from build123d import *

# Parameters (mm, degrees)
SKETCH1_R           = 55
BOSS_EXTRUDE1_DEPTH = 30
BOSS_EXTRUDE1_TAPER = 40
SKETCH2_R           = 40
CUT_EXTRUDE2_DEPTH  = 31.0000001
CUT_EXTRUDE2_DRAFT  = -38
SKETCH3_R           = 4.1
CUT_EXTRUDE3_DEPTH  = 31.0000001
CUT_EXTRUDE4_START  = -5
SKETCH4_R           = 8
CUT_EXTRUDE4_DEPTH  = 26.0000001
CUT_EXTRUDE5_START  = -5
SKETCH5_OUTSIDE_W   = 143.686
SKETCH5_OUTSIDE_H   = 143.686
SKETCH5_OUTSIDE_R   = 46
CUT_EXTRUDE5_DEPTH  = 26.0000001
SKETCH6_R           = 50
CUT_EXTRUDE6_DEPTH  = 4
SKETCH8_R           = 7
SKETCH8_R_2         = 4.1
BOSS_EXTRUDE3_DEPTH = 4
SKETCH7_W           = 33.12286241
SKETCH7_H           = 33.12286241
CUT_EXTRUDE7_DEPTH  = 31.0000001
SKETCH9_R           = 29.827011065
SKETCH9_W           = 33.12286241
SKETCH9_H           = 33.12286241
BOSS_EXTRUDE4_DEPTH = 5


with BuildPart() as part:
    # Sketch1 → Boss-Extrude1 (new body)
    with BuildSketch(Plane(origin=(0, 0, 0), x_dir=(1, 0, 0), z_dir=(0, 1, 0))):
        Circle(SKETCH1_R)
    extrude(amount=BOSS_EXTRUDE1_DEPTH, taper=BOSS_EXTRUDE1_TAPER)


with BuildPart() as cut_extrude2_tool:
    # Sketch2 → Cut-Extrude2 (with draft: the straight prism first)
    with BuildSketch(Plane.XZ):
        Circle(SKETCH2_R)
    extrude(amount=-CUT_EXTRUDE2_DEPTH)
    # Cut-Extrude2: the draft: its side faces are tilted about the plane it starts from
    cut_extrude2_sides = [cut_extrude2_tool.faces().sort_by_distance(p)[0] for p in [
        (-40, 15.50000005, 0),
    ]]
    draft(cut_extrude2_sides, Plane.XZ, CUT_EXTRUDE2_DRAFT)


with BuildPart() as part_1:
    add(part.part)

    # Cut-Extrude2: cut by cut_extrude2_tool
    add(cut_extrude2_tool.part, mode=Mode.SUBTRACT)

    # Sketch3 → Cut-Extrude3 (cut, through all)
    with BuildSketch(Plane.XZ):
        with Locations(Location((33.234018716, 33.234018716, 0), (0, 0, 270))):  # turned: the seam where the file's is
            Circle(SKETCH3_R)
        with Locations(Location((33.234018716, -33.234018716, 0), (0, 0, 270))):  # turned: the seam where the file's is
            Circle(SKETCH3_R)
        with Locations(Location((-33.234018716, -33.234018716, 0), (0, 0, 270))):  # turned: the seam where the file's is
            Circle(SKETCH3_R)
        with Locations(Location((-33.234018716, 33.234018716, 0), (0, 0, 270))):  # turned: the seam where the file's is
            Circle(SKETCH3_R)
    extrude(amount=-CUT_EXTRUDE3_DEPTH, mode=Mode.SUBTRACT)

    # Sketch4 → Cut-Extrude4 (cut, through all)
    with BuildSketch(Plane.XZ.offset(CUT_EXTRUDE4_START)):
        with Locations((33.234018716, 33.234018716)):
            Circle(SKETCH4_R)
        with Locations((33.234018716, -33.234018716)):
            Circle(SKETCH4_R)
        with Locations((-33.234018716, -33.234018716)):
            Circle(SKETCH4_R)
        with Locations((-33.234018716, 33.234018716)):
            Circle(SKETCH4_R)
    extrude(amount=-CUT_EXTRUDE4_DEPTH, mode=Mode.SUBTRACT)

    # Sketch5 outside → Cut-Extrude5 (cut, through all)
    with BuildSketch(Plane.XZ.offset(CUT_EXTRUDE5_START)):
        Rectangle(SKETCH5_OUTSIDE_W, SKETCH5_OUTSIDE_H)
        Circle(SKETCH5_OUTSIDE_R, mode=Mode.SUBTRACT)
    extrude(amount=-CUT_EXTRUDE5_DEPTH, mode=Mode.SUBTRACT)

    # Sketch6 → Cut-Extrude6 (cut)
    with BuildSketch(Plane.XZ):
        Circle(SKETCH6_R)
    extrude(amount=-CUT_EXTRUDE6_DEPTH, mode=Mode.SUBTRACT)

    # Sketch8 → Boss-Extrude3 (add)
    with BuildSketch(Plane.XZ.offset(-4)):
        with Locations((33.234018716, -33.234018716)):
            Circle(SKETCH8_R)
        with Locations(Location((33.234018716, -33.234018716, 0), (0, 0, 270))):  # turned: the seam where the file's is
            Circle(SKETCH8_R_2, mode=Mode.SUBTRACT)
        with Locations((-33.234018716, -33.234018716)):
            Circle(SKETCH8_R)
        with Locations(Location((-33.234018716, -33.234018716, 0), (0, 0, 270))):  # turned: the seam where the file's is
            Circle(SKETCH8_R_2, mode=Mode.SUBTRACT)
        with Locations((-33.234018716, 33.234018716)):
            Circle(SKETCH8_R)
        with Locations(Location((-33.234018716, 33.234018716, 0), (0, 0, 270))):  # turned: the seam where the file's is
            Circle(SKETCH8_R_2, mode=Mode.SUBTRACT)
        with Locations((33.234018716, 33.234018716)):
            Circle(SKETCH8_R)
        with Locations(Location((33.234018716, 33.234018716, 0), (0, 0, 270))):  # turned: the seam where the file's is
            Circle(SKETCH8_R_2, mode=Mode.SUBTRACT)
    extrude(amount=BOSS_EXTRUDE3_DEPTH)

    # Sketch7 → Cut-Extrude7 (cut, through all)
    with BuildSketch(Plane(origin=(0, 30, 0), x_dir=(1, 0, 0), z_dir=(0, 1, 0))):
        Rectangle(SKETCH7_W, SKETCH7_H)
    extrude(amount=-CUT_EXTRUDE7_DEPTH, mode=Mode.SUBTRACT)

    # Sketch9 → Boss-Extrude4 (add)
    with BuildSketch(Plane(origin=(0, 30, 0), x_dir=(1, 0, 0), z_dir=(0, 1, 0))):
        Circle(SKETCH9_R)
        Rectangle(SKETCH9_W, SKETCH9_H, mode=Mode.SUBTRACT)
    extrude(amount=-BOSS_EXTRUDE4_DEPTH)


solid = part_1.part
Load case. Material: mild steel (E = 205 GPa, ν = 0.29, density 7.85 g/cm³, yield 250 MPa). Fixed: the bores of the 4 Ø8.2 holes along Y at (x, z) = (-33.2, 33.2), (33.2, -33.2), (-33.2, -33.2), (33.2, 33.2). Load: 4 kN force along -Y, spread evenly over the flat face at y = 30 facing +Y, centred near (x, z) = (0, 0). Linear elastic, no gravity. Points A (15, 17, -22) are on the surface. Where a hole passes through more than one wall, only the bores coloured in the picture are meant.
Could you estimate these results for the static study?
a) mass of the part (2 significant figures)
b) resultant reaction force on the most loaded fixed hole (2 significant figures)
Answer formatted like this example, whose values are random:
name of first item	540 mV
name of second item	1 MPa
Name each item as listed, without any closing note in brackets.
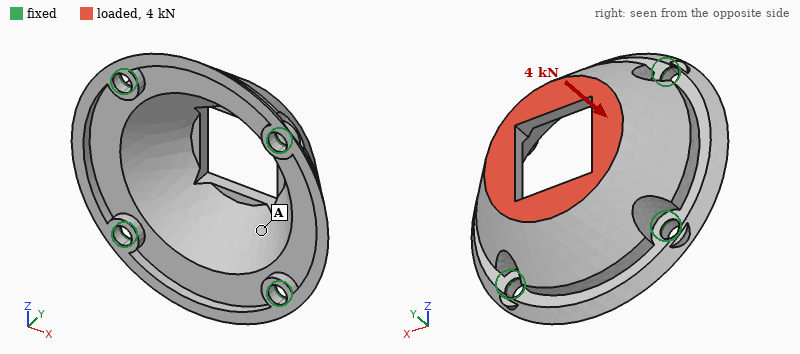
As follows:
mass of the part	590 g
resultant reaction force on the most loaded fixed hole	1.3 kN
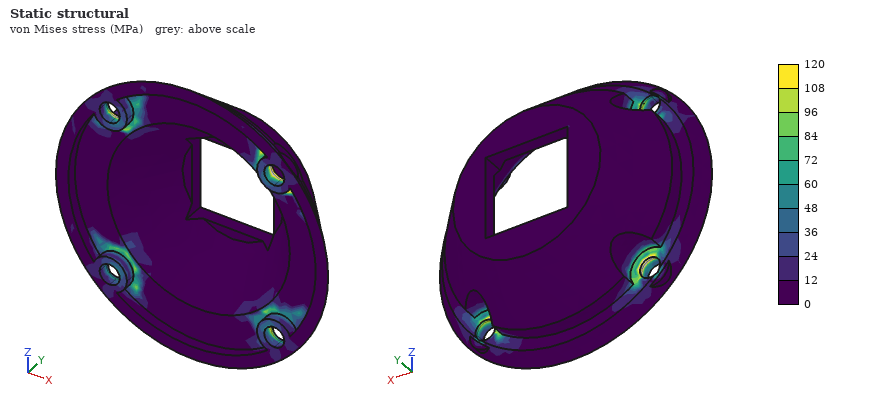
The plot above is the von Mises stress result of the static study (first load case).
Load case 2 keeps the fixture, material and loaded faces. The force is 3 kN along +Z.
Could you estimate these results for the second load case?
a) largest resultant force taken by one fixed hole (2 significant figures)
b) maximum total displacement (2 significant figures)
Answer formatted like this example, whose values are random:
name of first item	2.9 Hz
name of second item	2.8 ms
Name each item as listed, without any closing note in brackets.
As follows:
largest resultant force taken by one fixed hole	980 N
maximum total displacement	7.2 µm
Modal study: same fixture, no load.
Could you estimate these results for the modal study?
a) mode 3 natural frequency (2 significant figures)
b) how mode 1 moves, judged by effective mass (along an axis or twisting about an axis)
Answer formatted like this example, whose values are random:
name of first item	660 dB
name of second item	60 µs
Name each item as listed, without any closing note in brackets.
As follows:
mode 3 natural frequency	6300 Hz
how mode 1 moves, judged by effective mass	along Y
